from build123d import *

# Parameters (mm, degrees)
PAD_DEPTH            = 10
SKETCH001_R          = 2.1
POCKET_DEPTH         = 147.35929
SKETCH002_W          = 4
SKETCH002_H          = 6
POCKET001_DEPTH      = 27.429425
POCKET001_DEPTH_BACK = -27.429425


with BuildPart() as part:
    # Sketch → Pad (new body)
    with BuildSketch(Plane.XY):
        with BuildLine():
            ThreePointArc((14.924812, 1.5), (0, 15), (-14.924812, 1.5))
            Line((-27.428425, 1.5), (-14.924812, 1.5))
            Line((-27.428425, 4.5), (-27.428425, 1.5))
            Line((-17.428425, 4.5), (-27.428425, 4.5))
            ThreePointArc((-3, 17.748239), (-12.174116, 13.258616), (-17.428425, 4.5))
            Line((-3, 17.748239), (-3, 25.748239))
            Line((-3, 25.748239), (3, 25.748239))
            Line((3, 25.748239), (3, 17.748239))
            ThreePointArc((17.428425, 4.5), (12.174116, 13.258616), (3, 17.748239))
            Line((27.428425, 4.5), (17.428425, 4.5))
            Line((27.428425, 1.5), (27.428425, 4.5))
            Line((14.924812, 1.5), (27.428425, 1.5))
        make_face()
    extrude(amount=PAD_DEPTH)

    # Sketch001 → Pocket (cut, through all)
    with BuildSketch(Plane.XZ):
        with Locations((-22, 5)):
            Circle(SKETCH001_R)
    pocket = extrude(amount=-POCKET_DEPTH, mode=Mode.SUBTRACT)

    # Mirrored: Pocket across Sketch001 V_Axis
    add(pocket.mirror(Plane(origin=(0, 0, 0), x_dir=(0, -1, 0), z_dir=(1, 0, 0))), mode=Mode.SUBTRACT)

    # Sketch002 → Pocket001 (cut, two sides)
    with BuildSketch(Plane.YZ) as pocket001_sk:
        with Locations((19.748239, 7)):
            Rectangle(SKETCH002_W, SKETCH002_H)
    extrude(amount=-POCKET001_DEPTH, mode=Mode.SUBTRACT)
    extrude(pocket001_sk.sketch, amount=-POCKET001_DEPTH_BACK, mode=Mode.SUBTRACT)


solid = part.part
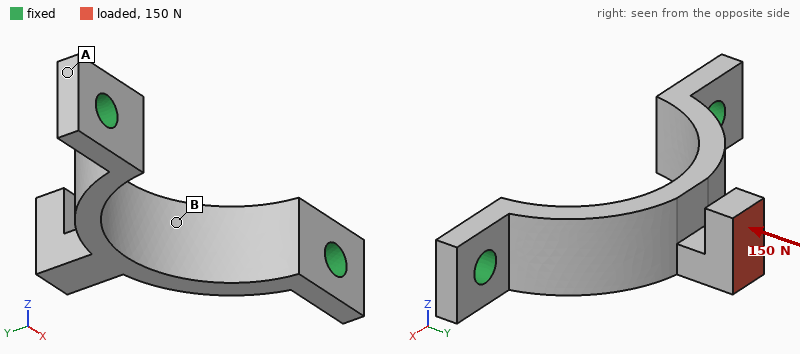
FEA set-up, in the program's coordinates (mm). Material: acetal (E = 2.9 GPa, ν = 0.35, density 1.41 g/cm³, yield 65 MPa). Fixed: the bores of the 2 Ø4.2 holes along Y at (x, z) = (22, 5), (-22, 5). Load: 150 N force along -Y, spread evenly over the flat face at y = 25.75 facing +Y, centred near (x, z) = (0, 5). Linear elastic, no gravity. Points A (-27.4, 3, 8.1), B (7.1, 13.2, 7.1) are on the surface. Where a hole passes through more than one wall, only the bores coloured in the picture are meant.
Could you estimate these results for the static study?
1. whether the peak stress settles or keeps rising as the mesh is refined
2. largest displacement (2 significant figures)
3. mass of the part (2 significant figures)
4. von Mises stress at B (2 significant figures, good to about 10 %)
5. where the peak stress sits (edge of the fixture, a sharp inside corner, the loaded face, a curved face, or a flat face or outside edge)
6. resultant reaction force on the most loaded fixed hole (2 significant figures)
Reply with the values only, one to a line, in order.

keeps rising
0.52 mm
3.2 g
7.9 MPa
a sharp inside corner
110 N
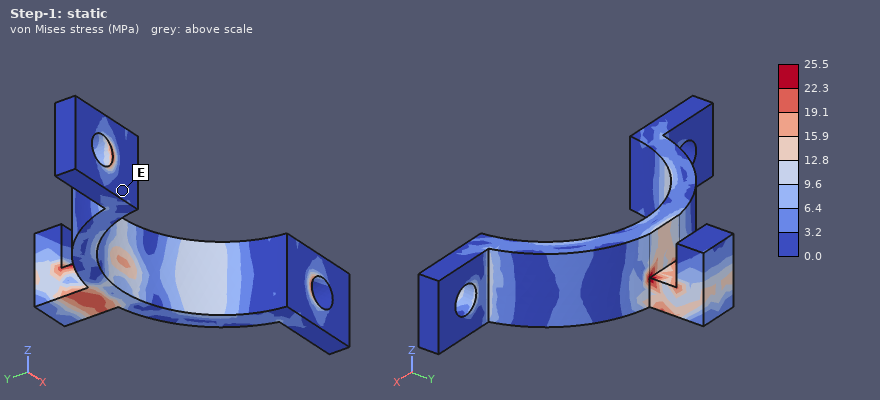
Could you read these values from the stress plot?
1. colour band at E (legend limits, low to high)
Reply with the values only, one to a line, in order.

0.0 to 3.2 MPa
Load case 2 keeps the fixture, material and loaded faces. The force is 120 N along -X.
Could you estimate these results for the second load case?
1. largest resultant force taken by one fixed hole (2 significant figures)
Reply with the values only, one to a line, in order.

97 N
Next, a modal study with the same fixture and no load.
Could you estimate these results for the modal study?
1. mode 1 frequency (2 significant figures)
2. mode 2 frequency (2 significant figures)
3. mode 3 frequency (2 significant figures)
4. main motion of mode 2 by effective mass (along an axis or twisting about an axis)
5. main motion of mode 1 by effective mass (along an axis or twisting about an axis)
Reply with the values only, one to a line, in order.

1500 Hz
3300 Hz
4400 Hz
along X
along Z
